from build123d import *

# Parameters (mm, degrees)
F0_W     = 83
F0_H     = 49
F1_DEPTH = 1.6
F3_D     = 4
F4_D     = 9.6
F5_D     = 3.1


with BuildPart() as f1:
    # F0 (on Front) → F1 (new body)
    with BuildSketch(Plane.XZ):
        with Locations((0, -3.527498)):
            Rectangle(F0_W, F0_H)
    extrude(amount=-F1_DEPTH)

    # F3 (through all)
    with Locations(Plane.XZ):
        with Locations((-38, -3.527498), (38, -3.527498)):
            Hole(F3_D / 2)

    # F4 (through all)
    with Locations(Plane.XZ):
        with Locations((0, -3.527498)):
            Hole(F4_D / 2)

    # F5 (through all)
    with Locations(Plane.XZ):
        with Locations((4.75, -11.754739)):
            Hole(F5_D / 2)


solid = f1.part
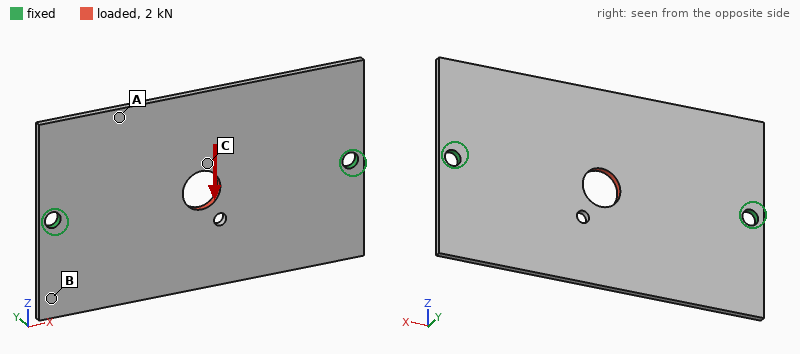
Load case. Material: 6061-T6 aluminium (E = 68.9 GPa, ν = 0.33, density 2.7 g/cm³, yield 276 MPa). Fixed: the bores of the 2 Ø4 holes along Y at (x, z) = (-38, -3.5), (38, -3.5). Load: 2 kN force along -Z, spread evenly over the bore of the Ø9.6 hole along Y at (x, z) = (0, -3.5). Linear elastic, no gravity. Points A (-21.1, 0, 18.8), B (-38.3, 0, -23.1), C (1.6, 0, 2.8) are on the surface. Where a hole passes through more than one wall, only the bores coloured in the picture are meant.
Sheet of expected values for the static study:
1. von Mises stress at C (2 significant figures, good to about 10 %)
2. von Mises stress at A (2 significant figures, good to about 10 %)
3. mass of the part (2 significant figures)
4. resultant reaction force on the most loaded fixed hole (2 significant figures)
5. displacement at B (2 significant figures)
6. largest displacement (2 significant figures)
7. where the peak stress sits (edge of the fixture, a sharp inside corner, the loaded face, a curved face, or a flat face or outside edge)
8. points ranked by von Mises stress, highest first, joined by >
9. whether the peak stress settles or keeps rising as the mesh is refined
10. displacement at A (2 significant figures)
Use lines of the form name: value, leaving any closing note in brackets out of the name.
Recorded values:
von Mises stress at C: 43 MPa
von Mises stress at A: 24 MPa
mass of the part: 17 g
resultant reaction force on the most loaded fixed hole: 1.0 kN
displacement at B: 13 µm
largest displacement: 42 µm
where the peak stress sits: edge of the fixture
points ranked by von Mises stress, highest first, joined by >: C > A > B
whether the peak stress settles or keeps rising as the mesh is refined: keeps rising
displacement at A: 25 µm
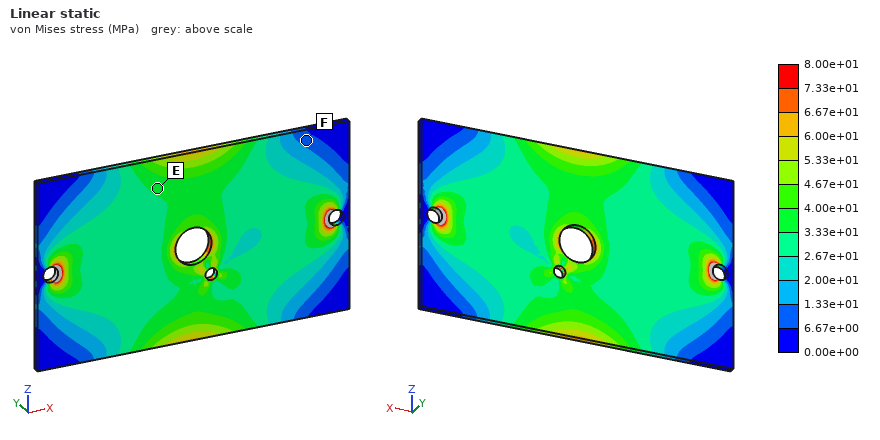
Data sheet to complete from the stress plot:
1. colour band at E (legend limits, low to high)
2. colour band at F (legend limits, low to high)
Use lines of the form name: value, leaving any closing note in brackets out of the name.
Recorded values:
colour band at E: 3.33e+01 to 4.00e+01 MPa
colour band at F: 6.67e+00 to 1.33e+01 MPa
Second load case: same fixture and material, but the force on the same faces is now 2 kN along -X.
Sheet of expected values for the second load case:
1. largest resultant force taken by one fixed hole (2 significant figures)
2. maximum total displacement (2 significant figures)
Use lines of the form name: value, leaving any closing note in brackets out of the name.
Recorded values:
largest resultant force taken by one fixed hole: 1.0 kN
maximum total displacement: 19 µm
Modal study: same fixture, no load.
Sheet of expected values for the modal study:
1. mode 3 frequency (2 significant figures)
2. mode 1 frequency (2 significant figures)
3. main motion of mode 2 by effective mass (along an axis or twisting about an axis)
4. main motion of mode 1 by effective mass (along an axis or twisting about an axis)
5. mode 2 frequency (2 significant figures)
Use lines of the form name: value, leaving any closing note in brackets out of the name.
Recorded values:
mode 3 frequency: 2300 Hz
mode 1 frequency: 1100 Hz
main motion of mode 2 by effective mass: along Y
main motion of mode 1 by effective mass: twisting about X
mode 2 frequency: 1100 Hz
